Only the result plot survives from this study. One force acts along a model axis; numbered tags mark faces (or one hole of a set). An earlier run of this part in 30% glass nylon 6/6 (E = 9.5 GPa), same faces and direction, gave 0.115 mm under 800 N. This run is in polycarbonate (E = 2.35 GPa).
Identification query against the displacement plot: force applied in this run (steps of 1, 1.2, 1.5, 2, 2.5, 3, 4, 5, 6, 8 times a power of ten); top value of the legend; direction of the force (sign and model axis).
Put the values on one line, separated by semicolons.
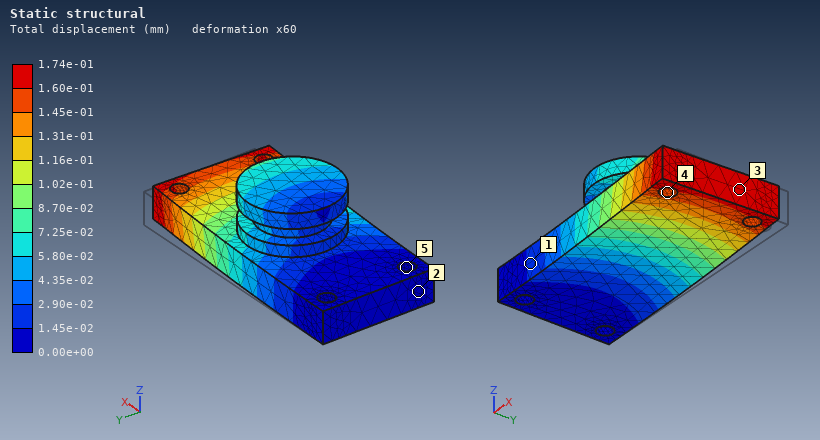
300 N; 1.74e-01 mm; -Y
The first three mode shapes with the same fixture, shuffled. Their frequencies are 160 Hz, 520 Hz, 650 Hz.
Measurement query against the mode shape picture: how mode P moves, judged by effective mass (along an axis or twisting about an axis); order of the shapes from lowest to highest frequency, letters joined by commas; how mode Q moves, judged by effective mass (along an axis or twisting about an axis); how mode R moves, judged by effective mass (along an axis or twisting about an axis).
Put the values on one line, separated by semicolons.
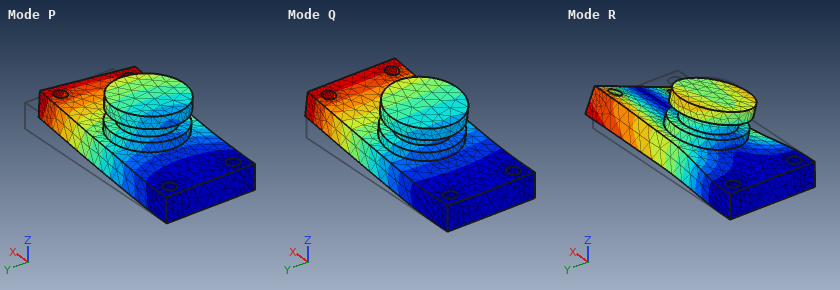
along Y; Q, P, R; along Z; twisting about X
